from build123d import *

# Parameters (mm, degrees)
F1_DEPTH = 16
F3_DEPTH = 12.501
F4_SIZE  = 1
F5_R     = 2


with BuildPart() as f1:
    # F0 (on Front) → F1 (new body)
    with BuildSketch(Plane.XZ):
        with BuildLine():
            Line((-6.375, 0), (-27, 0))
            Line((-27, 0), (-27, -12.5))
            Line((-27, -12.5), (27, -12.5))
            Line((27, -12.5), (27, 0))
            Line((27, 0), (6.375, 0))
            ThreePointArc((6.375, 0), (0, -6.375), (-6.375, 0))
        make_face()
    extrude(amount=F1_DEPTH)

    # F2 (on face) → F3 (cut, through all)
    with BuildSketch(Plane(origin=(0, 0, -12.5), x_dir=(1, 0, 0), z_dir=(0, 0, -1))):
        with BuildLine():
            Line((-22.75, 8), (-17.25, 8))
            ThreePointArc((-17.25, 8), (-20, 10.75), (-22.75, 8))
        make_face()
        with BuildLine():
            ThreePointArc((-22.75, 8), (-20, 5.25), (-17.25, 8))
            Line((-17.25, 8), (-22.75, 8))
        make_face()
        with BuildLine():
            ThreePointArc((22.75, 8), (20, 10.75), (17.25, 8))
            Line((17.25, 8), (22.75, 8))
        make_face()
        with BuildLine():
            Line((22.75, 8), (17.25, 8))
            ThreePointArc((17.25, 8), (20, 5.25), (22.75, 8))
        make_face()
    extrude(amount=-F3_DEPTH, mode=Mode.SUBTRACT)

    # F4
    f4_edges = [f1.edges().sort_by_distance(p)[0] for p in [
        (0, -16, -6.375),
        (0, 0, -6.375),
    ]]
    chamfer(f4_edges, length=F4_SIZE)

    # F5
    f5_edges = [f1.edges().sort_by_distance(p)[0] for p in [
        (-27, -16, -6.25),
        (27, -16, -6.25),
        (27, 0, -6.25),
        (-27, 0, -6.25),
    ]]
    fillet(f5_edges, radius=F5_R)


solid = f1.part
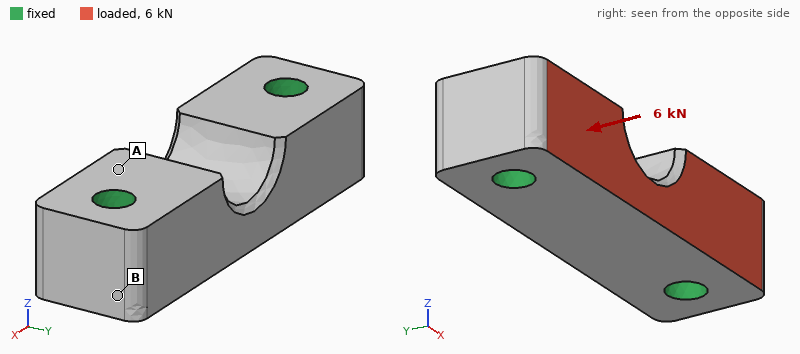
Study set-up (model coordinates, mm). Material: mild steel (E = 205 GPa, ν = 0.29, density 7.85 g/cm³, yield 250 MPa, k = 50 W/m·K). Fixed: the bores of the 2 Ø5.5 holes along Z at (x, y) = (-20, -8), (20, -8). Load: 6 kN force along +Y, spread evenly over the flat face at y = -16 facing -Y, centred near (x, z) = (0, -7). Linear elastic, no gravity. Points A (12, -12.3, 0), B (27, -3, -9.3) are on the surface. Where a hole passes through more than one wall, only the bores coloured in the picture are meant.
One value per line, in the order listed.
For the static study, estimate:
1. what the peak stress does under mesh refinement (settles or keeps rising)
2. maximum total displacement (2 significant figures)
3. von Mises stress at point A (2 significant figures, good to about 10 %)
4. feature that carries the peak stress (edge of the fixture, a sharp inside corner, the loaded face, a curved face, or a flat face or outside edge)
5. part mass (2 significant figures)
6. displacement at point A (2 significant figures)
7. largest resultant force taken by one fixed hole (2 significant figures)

keeps rising
3.8 µm
12 MPa
edge of the fixture
72 g
1.6 µm
3.0 kN
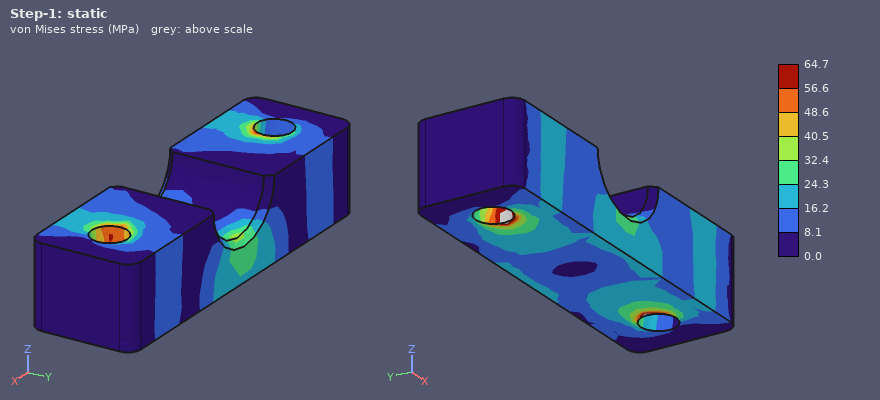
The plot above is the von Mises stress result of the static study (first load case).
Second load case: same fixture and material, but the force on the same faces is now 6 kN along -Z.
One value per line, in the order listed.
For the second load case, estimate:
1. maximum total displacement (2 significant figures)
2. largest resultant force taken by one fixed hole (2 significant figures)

7.7 µm
3.0 kN
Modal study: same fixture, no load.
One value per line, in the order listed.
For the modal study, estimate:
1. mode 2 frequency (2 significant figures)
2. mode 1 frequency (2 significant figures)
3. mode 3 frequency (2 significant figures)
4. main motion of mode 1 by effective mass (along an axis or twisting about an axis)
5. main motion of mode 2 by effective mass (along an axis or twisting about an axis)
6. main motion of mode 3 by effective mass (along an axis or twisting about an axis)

30 kHz
28 kHz
44 kHz
along Y
along Z
twisting about X
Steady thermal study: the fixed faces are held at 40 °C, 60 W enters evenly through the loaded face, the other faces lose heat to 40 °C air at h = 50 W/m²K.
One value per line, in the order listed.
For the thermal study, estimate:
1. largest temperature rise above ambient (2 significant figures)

32 K
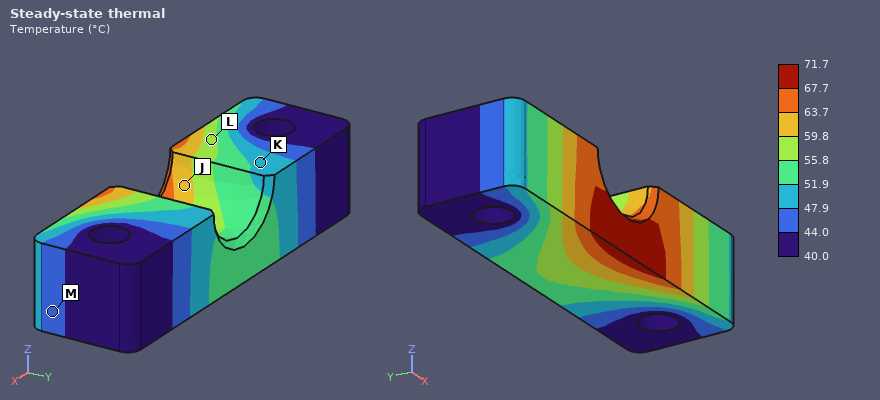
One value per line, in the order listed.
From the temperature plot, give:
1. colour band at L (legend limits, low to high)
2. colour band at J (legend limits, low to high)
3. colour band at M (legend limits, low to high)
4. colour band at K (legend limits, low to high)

55.8 to 59.8 °C
59.8 to 63.7 °C
44.0 to 47.9 °C
47.9 to 51.9 °C
